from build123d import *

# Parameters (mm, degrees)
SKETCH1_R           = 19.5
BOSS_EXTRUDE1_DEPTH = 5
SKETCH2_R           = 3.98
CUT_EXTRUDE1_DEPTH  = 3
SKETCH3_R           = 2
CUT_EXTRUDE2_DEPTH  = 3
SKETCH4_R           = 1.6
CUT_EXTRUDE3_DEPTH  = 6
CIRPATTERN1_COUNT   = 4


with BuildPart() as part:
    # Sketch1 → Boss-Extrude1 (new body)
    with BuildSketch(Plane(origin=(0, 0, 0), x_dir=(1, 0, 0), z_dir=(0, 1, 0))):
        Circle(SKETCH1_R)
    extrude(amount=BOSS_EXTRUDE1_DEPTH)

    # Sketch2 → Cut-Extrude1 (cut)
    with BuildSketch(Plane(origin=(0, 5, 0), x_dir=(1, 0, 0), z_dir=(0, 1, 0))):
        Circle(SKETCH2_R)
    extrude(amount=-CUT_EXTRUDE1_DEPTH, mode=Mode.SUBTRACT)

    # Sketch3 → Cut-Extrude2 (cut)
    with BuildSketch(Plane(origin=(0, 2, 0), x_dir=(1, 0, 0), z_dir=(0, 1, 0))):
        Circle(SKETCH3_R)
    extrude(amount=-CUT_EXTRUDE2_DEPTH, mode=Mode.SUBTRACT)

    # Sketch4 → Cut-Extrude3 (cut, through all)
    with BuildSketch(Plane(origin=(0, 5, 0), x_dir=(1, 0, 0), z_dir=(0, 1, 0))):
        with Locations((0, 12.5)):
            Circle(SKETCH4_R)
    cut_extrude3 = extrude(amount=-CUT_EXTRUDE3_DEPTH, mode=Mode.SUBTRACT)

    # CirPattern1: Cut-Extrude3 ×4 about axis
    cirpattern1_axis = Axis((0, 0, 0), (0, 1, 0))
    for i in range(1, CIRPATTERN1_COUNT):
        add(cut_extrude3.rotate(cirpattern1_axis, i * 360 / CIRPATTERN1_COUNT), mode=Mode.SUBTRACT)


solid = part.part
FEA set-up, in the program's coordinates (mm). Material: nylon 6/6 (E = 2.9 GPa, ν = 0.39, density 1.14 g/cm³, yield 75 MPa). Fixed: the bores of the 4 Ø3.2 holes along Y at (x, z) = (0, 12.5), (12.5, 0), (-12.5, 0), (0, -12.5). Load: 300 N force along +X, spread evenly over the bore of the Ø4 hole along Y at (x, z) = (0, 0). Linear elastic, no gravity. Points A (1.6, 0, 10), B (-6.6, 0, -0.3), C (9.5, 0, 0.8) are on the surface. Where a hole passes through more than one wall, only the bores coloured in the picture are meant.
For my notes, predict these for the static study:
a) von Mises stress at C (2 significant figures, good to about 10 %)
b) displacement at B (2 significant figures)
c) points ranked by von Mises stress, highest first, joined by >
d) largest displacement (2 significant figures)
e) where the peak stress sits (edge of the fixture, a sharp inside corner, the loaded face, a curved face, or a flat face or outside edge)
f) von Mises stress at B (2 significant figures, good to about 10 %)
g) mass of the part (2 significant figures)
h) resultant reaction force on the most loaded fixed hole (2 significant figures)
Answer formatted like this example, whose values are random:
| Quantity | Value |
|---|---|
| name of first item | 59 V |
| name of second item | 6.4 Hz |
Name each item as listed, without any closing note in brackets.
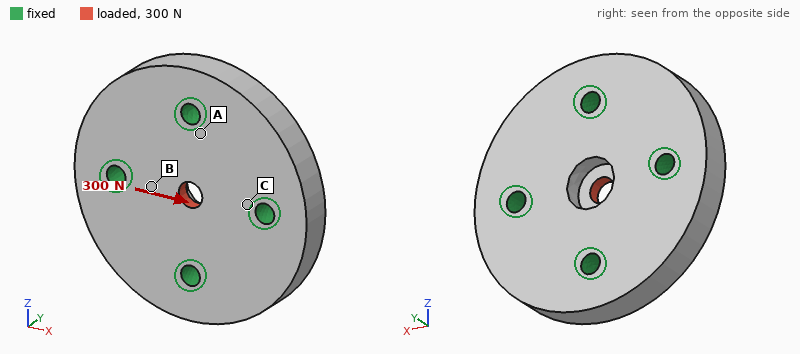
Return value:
| Quantity | Value |
|---|---|
| von Mises stress at C | 4.4 MPa |
| displacement at B | 7.7 µm |
| points ranked by von Mises stress, highest first, joined by > | B > C > A |
| largest displacement | 23 µm |
| where the peak stress sits | the loaded face |
| von Mises stress at B | 6.5 MPa |
| mass of the part | 6.4 g |
| resultant reaction force on the most loaded fixed hole | 100 N |
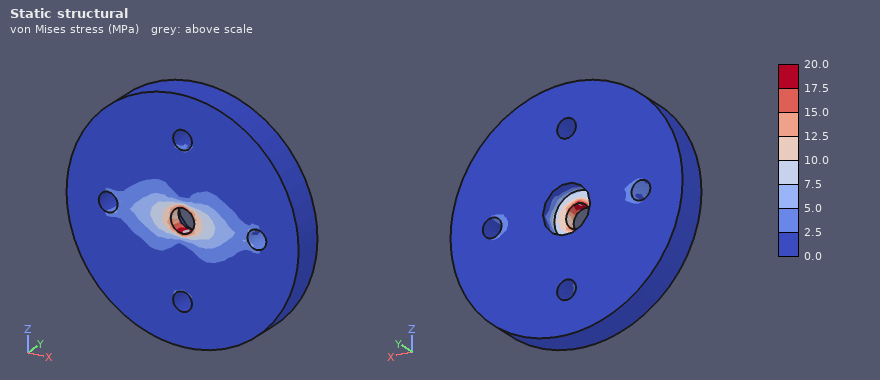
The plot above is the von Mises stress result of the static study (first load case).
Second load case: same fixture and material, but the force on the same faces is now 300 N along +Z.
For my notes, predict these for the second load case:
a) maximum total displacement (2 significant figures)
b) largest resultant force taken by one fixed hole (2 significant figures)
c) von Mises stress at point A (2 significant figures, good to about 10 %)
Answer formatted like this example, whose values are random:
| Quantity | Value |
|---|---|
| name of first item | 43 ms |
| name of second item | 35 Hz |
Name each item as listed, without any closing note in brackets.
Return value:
| Quantity | Value |
|---|---|
| maximum total displacement | 23 µm |
| largest resultant force taken by one fixed hole | 100 N |
| von Mises stress at point A | 3.2 MPa |
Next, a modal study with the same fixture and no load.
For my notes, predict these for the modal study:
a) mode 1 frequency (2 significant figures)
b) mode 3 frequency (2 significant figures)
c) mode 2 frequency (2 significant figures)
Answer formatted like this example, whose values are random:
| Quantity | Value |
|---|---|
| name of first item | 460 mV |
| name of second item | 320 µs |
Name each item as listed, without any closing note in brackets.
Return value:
| Quantity | Value |
|---|---|
| mode 1 frequency | 10000 Hz |
| mode 3 frequency | 11 kHz |
| mode 2 frequency | 11 kHz |
